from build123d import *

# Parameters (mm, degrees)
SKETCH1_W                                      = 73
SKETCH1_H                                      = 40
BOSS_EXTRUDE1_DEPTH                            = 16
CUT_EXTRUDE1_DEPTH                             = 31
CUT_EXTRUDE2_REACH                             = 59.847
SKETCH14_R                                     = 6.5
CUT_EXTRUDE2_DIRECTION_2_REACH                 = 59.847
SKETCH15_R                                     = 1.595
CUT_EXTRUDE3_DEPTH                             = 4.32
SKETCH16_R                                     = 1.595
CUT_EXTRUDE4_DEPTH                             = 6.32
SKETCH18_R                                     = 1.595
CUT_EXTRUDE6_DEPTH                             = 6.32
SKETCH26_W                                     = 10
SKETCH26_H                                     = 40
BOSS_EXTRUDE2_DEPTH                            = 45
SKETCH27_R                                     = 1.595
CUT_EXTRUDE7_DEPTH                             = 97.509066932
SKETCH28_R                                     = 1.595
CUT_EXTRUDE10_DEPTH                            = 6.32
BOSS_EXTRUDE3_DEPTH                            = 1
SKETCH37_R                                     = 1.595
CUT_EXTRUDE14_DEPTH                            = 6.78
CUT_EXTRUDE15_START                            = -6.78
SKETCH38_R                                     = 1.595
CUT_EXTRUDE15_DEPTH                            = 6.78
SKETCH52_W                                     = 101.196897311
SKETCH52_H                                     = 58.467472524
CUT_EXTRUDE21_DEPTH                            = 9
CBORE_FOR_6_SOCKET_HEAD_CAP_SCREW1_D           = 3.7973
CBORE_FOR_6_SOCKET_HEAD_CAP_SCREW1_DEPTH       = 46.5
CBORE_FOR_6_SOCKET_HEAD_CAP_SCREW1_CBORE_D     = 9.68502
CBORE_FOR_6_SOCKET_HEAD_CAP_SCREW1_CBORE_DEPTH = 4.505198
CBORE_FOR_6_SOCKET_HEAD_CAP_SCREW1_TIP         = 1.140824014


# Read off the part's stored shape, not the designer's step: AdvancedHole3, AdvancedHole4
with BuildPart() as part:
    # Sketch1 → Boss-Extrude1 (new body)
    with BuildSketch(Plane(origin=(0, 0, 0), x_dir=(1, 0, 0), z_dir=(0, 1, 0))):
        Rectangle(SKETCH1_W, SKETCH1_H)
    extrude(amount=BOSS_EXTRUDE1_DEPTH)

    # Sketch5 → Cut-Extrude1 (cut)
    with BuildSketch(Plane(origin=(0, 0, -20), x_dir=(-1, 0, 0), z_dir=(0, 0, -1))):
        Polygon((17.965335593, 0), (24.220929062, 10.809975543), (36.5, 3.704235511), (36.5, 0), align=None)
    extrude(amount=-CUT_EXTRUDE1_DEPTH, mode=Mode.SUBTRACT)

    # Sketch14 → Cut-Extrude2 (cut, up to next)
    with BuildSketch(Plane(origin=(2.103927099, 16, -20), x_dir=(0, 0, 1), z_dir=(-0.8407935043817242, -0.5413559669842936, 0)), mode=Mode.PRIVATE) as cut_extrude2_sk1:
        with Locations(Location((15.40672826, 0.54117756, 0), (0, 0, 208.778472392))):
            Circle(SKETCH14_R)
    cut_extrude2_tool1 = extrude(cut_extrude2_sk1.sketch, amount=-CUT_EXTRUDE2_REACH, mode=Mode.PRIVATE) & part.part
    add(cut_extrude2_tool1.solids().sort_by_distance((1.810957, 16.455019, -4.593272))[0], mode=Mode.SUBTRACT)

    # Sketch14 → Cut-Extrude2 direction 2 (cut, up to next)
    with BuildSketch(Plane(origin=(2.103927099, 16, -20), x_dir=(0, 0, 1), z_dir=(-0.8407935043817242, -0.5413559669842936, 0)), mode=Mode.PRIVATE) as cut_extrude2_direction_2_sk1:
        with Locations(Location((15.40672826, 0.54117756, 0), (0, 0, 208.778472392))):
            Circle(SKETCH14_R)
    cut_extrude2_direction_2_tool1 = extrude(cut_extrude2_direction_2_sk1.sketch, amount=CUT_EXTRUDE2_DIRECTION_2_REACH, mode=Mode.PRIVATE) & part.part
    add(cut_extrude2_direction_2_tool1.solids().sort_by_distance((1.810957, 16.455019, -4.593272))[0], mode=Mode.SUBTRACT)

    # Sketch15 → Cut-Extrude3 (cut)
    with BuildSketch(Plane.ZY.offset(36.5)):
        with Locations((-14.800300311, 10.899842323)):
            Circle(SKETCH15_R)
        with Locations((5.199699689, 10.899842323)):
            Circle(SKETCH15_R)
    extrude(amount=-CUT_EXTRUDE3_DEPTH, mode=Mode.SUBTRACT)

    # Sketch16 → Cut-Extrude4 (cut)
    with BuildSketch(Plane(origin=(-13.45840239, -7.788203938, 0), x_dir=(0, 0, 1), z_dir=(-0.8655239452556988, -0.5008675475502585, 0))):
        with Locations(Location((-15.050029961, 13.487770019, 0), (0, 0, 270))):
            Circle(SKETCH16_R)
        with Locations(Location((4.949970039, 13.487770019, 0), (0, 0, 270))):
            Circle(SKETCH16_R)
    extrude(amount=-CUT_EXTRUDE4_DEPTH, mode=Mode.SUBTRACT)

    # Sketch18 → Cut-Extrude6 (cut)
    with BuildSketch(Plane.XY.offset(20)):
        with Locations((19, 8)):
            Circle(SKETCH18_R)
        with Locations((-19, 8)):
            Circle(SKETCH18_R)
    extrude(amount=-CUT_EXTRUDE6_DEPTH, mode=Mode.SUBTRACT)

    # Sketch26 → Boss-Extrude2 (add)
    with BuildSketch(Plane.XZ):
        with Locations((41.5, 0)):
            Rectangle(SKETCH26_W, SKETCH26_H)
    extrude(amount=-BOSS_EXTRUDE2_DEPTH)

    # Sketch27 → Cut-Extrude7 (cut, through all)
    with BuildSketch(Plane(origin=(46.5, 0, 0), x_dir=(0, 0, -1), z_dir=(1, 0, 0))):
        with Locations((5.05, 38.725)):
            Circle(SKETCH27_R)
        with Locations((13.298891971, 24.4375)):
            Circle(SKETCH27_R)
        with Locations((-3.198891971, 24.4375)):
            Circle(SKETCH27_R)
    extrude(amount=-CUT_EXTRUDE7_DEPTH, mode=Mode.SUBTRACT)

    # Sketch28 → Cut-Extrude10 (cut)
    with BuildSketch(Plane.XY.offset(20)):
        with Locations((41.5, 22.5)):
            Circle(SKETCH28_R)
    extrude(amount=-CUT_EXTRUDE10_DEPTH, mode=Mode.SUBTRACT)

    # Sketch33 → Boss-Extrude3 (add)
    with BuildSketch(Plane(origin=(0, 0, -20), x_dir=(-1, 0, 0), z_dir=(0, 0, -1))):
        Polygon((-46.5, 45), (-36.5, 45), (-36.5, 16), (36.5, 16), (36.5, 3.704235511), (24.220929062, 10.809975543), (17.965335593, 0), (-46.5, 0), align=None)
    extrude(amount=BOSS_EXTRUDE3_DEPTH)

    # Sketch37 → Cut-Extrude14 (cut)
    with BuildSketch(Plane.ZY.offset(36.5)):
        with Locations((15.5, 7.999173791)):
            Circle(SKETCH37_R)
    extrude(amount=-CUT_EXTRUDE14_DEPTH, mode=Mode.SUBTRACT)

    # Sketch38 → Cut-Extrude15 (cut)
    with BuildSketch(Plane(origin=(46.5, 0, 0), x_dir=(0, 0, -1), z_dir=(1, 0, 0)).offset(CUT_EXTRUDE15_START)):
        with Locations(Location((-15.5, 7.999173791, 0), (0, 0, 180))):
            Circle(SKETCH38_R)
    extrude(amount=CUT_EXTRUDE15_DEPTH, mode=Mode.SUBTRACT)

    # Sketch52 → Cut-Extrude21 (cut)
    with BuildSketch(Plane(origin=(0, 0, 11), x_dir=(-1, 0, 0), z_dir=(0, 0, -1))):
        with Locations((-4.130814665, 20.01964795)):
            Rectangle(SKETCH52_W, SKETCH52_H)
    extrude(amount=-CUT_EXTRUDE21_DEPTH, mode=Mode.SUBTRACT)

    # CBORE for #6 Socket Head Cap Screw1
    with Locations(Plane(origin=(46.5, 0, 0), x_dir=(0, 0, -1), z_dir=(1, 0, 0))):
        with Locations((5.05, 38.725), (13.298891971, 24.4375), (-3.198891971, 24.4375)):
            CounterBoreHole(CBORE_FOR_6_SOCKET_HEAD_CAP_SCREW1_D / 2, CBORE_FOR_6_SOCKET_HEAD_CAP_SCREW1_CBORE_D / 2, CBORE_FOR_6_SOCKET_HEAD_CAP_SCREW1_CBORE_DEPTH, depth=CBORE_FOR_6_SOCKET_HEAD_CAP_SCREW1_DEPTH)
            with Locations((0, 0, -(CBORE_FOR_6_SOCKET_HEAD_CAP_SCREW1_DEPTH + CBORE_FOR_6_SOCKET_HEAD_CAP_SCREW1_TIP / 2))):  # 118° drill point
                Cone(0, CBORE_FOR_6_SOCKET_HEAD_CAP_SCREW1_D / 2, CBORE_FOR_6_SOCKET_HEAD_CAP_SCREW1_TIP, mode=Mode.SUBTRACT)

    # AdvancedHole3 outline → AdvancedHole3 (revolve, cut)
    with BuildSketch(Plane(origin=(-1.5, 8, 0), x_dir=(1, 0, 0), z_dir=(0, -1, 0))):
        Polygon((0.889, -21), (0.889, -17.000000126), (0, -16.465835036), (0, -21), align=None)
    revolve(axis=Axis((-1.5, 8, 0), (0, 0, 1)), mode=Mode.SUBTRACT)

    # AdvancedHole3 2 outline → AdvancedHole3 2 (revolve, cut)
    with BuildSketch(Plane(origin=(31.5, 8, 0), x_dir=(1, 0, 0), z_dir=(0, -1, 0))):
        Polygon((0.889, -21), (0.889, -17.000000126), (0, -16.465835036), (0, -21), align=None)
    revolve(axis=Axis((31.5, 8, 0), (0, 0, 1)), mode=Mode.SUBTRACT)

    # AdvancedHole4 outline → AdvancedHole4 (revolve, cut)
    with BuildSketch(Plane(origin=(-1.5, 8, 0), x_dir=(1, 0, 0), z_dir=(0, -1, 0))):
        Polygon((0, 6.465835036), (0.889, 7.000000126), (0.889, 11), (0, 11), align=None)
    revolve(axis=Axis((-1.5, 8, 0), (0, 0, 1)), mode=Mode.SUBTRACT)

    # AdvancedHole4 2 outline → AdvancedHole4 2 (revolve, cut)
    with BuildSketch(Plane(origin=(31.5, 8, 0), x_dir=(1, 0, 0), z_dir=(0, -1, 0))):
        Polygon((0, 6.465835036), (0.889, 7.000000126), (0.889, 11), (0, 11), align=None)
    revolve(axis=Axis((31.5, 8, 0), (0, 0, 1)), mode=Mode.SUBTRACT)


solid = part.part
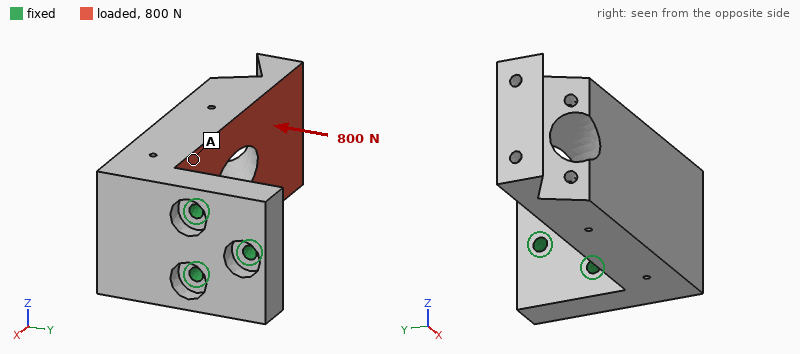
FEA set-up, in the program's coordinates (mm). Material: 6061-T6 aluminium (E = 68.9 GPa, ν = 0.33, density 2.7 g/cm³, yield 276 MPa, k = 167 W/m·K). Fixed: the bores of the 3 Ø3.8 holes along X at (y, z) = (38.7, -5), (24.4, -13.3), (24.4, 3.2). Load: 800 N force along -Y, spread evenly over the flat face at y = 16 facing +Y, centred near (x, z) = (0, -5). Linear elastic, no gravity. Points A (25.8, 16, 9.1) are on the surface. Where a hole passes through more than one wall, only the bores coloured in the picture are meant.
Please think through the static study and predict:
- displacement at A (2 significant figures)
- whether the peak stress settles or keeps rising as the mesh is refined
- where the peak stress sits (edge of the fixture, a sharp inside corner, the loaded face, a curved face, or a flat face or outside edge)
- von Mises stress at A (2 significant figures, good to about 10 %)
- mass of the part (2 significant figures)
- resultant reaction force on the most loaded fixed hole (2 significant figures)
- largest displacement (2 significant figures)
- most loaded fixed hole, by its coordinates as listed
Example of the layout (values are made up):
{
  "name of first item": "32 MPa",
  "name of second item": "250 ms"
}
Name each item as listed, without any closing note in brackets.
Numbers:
{
  "displacement at A": "0.059 mm",
  "whether the peak stress settles or keeps rising as the mesh is refined": "keeps rising",
  "where the peak stress sits": "edge of the fixture",
  "von Mises stress at A": "14 MPa",
  "mass of the part": "120 g",
  "resultant reaction force on the most loaded fixed hole": "1.3 kN",
  "largest displacement": "0.37 mm",
  "most loaded fixed hole, by its coordinates as listed": "(38.7, -5)"
}
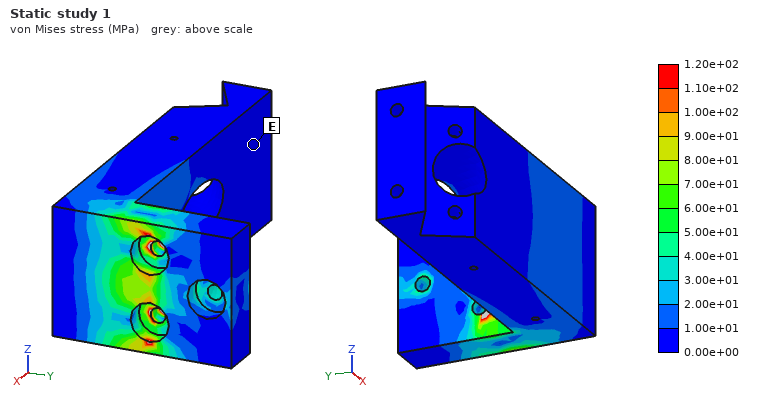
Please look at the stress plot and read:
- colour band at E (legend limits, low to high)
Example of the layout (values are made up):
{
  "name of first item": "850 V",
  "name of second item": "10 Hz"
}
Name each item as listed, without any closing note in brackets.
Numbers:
{
  "colour band at E": "0.00e+00 to 1.00e+01 MPa"
}
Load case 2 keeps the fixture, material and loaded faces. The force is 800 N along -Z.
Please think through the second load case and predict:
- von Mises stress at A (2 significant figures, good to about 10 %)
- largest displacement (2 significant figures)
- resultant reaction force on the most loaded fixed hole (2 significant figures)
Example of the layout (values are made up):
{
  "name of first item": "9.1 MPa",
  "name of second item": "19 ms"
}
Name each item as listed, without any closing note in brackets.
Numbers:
{
  "von Mises stress at A": "12 MPa",
  "largest displacement": "0.13 mm",
  "resultant reaction force on the most loaded fixed hole": "1.6 kN"
}
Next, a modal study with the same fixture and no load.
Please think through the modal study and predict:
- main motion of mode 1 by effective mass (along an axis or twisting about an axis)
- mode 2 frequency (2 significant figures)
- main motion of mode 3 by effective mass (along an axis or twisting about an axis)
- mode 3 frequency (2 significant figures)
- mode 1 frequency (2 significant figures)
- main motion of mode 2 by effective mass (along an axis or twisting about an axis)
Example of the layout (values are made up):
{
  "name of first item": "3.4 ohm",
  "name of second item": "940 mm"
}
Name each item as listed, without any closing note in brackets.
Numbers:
{
  "main motion of mode 1 by effective mass": "along Y",
  "mode 2 frequency": "1900 Hz",
  "main motion of mode 3 by effective mass": "along X",
  "mode 3 frequency": "5900 Hz",
  "mode 1 frequency": "1100 Hz",
  "main motion of mode 2 by effective mass": "along Z"
}
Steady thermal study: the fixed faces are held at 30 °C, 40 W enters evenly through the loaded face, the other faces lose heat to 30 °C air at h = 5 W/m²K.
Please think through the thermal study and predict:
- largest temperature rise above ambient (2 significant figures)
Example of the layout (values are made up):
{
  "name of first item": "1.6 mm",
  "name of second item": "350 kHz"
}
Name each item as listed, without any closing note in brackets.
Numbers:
{
  "largest temperature rise above ambient": "35 K"
}
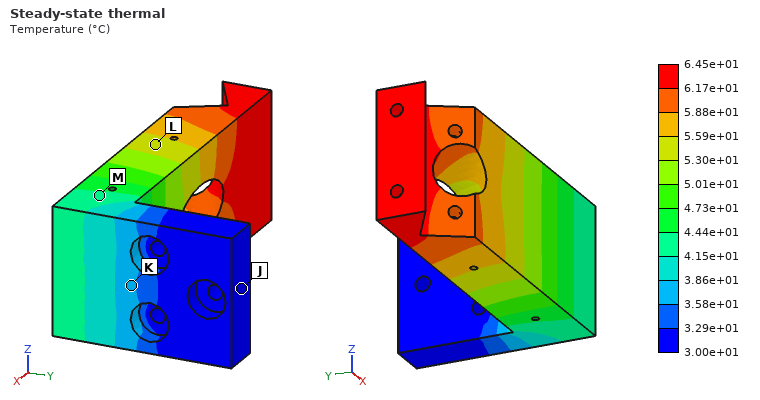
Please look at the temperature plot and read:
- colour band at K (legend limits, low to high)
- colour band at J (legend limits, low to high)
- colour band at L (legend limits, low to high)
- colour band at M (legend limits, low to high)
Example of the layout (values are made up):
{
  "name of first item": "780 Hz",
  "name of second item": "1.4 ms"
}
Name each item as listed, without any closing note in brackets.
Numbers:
{
  "colour band at K": "3.58e+01 to 3.86e+01 °C",
  "colour band at J": "3.00e+01 to 3.29e+01 °C",
  "colour band at L": "5.30e+01 to 5.59e+01 °C",
  "colour band at M": "4.15e+01 to 4.44e+01 °C"
}
